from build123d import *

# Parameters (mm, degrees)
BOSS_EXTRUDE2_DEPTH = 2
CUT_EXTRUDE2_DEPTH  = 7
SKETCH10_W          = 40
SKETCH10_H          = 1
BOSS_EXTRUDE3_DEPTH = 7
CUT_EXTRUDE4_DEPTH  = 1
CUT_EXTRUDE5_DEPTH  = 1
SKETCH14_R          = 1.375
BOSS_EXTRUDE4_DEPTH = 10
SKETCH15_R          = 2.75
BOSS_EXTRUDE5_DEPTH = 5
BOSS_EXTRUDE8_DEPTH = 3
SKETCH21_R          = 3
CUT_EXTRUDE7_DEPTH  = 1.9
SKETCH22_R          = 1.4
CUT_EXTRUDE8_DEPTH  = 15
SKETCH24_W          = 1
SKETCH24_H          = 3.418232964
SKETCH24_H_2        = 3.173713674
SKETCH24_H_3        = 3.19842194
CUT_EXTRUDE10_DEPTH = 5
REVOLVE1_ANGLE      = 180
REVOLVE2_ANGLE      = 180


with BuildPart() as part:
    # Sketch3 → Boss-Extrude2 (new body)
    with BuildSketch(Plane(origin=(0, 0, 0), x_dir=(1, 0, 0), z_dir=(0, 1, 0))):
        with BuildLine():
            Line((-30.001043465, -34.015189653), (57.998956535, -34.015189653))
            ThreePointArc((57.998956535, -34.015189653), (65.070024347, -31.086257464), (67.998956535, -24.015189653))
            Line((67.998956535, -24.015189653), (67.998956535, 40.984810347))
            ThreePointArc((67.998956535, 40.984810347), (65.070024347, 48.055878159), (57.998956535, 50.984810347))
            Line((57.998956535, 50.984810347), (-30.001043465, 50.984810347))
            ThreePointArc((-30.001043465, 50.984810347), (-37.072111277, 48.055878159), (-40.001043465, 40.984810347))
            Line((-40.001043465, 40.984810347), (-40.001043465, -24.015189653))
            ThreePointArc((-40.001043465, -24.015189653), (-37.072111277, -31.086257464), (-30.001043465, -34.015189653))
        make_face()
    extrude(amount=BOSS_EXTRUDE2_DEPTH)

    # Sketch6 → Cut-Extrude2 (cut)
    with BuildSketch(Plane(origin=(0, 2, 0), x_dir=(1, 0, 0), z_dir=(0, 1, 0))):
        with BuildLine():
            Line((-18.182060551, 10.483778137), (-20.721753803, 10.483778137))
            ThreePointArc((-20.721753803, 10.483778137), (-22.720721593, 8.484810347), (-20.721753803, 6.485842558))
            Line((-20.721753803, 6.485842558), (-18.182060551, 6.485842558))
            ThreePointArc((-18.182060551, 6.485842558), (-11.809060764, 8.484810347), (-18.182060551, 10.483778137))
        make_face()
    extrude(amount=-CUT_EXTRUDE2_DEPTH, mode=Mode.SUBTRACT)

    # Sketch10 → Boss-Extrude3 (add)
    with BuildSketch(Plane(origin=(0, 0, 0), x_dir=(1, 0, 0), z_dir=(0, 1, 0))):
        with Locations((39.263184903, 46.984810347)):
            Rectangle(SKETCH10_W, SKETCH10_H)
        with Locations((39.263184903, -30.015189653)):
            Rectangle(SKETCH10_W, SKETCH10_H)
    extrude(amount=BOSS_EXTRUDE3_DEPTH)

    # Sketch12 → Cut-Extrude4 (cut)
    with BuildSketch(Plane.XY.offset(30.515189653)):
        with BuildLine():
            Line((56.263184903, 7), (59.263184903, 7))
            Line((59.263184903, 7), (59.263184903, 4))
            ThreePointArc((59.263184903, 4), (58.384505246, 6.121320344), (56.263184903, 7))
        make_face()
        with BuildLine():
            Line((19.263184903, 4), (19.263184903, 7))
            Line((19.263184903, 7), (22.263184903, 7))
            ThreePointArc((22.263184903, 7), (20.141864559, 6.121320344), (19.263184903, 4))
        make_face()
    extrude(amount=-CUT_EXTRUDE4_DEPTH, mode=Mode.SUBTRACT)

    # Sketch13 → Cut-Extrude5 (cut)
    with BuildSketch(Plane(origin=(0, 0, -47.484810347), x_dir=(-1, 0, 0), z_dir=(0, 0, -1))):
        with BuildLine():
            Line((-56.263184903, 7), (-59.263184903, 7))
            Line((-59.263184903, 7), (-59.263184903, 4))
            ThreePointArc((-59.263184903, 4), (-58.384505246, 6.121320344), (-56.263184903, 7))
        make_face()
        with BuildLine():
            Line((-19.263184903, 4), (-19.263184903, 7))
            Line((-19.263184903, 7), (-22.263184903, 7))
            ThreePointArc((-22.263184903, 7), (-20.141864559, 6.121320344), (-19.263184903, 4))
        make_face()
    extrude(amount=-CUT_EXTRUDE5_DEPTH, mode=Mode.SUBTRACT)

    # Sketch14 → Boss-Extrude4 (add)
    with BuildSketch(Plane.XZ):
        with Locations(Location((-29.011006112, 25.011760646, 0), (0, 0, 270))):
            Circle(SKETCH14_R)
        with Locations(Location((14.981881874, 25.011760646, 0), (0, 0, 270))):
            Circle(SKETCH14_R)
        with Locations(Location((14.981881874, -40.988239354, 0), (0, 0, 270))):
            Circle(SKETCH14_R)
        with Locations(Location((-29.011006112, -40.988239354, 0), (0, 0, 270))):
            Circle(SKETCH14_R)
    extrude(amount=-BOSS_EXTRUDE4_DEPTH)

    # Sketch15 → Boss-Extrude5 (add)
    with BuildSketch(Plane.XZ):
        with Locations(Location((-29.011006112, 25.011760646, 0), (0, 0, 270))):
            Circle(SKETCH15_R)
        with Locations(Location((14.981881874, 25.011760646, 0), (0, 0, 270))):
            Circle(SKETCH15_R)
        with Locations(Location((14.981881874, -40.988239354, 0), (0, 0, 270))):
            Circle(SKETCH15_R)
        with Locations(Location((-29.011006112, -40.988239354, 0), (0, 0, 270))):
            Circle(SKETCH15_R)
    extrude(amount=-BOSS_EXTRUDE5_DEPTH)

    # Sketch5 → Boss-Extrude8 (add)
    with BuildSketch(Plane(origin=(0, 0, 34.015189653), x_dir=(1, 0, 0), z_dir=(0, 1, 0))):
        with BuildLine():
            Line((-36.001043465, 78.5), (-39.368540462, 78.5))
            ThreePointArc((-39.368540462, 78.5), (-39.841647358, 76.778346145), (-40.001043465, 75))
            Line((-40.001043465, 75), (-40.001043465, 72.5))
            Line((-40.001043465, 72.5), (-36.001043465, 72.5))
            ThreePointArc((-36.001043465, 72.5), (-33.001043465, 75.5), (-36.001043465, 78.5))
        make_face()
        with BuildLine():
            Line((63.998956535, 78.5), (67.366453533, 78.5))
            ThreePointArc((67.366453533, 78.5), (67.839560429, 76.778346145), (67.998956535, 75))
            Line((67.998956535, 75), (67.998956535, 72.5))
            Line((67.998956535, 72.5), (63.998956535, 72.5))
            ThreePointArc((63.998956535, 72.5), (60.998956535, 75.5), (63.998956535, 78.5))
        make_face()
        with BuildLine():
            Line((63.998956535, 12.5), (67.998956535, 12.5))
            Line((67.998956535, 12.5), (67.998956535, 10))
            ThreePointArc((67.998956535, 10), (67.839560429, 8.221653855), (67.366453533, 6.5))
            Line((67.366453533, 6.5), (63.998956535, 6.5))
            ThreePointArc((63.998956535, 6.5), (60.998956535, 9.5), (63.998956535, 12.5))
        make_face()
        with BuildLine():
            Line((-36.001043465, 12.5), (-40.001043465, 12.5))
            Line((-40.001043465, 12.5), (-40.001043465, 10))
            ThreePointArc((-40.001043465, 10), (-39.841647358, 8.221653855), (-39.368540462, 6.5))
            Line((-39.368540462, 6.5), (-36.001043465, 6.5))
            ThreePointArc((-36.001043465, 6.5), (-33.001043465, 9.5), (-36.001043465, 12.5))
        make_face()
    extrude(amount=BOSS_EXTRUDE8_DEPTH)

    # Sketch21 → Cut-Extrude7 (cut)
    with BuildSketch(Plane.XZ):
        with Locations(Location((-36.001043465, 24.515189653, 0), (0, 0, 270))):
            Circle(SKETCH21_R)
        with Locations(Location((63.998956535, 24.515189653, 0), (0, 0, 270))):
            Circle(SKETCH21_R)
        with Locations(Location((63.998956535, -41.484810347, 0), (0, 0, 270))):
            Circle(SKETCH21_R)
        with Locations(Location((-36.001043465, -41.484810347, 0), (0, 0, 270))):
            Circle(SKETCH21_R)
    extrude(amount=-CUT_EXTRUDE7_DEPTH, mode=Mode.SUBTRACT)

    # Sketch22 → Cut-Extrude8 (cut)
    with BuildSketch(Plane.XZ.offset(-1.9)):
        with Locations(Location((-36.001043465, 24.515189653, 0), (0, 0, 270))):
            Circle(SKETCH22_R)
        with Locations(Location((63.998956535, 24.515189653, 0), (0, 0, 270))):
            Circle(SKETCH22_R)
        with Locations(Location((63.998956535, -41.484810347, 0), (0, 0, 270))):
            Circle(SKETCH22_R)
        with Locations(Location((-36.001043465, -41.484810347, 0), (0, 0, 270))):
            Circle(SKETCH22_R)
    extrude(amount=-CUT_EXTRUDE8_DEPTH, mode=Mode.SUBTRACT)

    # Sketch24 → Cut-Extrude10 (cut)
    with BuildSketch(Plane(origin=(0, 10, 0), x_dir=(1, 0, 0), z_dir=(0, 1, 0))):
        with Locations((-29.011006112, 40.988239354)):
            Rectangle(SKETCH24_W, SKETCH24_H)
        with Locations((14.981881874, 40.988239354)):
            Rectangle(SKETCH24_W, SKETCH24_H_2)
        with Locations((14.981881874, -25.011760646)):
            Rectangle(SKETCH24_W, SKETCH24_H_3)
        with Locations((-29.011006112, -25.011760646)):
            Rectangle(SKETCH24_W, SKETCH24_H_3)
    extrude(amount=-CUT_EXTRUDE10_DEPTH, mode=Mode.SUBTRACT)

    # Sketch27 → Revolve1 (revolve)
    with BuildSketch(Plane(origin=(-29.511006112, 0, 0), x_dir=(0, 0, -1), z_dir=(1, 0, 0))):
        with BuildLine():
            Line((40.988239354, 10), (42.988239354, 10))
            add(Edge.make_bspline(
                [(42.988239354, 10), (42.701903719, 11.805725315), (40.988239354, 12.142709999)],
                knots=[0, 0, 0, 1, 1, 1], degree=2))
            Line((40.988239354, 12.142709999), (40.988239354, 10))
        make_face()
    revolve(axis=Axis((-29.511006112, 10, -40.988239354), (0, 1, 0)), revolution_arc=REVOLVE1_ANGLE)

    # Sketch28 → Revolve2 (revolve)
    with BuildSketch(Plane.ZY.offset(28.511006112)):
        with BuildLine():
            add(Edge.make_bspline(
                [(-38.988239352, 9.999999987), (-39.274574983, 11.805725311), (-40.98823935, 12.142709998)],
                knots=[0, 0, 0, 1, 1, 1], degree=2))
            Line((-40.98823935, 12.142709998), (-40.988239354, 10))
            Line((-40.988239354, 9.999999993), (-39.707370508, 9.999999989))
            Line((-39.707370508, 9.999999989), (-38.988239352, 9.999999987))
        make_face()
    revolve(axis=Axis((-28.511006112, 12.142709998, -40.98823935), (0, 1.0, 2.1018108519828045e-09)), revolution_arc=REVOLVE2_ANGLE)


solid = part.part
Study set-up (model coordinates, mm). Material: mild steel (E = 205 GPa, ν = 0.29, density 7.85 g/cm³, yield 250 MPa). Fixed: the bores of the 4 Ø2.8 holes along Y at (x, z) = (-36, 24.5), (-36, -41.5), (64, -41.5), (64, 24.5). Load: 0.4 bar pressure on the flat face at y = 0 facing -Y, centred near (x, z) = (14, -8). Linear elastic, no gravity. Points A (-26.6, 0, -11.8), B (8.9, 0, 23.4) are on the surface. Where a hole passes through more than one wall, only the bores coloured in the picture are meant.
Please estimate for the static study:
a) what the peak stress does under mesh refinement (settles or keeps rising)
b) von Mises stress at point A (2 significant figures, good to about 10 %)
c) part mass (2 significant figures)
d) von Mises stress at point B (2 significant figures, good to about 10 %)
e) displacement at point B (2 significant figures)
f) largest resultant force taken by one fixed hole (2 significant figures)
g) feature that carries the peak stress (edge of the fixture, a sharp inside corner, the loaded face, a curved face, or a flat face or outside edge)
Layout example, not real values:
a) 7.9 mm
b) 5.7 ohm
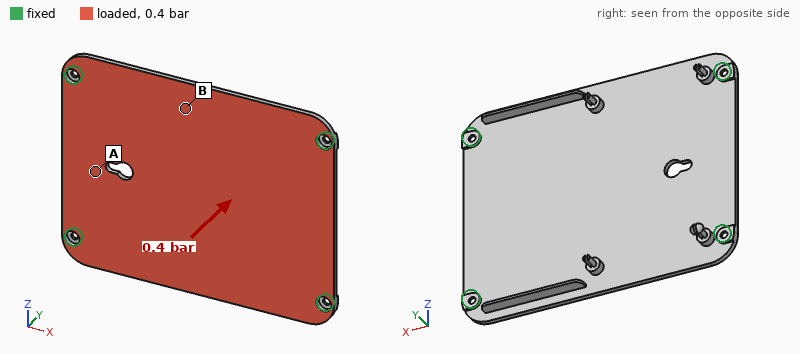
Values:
a) keeps rising
b) 23 MPa
c) 150 g
d) 39 MPa
e) 0.12 mm
f) 350 N
g) a sharp inside corner
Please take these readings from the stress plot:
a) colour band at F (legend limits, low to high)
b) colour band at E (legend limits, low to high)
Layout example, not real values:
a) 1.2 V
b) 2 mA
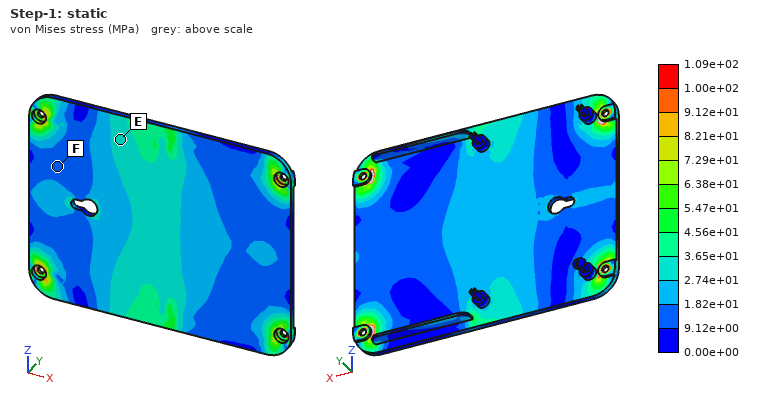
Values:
a) 9.12e+00 to 1.82e+01 MPa
b) 2.74e+01 to 3.65e+01 MPa
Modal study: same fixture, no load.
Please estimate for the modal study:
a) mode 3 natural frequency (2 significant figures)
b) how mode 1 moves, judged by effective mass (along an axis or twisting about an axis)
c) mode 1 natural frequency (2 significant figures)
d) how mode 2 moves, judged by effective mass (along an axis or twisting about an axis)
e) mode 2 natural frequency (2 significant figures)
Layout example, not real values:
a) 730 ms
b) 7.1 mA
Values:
a) 1900 Hz
b) along Y
c) 810 Hz
d) twisting about X
e) 1200 Hz
